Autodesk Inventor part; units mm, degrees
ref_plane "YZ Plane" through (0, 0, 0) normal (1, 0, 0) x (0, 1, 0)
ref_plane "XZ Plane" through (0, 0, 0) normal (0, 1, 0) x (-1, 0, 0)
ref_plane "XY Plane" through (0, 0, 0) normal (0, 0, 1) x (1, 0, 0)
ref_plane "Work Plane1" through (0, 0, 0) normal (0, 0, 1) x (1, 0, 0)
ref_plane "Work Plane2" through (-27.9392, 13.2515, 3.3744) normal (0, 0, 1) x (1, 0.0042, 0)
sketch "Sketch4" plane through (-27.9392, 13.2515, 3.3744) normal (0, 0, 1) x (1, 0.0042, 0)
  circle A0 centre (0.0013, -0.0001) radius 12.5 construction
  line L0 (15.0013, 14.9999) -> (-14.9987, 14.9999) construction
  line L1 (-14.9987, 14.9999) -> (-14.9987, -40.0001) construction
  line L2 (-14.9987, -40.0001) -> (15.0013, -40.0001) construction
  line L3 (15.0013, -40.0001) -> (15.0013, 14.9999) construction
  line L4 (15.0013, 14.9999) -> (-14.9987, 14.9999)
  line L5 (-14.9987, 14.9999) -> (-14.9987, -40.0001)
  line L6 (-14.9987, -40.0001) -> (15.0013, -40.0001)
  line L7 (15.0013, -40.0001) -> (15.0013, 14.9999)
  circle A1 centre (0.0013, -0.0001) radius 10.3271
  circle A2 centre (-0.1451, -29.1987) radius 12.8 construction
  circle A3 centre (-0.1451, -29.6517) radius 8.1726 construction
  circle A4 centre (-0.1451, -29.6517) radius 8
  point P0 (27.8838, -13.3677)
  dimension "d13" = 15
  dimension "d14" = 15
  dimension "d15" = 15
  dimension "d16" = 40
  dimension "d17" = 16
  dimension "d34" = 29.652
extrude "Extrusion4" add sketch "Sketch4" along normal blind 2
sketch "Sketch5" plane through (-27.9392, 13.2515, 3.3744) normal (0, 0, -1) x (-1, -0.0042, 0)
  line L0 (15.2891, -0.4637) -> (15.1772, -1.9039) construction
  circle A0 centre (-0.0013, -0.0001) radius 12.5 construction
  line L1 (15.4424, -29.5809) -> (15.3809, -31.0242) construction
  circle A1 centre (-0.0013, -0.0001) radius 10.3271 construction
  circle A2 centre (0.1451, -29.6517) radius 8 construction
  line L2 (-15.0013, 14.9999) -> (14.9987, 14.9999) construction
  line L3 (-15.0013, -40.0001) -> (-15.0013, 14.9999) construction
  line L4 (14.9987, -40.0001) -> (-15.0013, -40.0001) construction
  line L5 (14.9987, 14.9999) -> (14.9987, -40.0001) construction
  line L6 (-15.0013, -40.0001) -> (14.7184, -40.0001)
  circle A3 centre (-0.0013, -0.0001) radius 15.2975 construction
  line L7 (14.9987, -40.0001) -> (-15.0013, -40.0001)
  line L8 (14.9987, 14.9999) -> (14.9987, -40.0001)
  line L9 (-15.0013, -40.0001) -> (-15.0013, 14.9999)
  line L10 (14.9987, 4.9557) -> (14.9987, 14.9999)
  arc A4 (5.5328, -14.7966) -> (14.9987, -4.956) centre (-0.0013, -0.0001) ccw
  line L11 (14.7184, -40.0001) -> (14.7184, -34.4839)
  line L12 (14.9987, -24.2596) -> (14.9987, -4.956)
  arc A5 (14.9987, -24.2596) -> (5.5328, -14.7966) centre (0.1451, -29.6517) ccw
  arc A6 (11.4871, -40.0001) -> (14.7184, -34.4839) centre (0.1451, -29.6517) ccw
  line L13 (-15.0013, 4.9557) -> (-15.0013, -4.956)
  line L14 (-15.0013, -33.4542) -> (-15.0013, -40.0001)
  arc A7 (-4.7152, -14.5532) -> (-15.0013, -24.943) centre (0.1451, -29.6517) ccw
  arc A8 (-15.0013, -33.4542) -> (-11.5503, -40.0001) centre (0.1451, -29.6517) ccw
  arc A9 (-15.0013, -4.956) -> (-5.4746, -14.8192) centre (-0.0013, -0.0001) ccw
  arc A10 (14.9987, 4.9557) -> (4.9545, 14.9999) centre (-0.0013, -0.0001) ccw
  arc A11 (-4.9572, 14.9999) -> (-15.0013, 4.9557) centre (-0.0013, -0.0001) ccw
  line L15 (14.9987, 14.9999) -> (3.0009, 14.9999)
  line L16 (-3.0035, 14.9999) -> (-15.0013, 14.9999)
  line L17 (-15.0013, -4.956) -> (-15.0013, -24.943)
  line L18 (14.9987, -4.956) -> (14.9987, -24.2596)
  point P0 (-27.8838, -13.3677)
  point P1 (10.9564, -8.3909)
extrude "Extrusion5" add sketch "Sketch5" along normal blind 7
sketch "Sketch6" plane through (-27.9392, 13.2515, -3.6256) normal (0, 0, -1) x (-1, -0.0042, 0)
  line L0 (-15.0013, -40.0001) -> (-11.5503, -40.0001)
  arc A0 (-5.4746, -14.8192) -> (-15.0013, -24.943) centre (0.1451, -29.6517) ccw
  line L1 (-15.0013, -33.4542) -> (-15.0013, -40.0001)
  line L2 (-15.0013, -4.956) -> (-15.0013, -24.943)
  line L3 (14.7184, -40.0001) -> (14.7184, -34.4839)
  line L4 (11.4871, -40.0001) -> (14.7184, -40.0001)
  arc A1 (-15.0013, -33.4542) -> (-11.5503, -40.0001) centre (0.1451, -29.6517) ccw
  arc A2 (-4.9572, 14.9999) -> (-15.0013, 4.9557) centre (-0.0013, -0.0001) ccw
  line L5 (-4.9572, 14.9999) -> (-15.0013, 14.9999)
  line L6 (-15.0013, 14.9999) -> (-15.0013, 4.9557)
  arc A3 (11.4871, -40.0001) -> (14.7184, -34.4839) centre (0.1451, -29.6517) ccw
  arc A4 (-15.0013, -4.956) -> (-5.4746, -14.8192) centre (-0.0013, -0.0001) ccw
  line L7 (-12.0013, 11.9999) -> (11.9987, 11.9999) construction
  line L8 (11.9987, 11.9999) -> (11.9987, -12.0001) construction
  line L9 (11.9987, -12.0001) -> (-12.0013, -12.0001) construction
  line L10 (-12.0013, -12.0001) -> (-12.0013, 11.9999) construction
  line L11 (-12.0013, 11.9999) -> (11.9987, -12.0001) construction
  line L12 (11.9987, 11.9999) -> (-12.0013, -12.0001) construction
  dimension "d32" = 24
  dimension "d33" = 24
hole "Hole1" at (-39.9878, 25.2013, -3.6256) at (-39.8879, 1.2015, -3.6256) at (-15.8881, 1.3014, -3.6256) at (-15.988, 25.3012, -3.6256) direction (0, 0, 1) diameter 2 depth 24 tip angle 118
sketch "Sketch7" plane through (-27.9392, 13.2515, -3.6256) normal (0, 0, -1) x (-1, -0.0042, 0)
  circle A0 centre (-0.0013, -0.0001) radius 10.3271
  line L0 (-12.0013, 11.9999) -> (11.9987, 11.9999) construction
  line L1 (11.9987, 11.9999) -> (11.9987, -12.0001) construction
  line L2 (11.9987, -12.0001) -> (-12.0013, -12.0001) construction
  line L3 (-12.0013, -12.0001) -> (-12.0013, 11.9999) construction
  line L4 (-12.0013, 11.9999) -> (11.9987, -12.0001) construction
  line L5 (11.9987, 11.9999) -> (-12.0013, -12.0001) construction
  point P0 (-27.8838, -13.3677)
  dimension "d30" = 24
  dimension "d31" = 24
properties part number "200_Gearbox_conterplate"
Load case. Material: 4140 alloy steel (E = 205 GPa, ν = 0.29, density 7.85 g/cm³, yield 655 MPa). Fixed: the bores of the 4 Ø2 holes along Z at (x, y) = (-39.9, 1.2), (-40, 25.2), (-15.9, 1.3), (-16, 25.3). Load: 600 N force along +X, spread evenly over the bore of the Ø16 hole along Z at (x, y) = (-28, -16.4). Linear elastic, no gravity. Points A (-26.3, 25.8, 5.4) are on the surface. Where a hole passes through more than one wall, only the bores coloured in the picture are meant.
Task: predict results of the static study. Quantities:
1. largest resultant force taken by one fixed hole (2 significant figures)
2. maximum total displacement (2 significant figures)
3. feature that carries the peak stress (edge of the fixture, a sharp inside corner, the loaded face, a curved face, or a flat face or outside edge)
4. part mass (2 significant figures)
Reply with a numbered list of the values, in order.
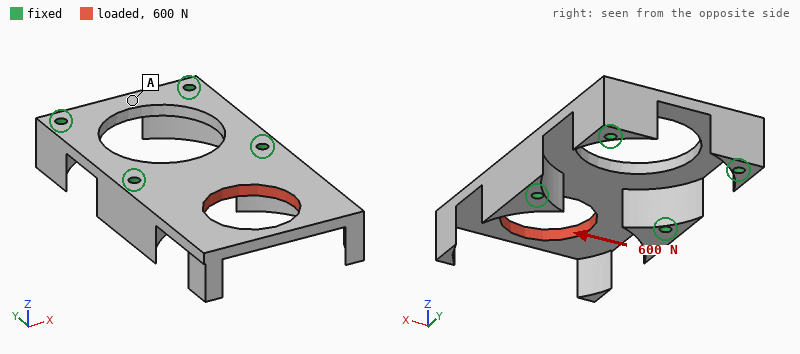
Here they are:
1. 480 N
2. 16 µm
3. the loaded face
4. 28 g
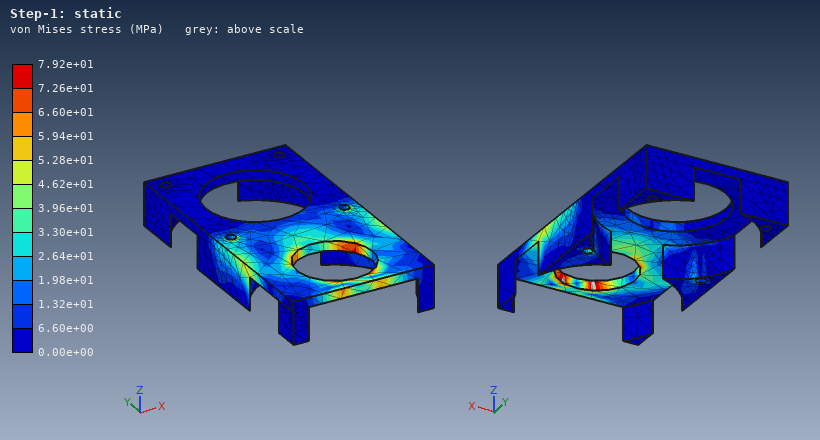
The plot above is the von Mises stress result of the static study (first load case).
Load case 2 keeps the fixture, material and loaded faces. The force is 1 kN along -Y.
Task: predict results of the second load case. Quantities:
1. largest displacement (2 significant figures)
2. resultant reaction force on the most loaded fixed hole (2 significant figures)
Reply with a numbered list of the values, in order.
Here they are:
1. 9.1 µm
2. 500 N
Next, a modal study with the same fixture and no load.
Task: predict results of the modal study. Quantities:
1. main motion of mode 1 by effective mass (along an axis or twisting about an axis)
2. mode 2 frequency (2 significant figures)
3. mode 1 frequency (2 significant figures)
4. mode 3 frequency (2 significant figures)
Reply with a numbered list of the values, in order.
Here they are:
1. along Z
2. 4900 Hz
3. 2900 Hz
4. 9700 Hz
